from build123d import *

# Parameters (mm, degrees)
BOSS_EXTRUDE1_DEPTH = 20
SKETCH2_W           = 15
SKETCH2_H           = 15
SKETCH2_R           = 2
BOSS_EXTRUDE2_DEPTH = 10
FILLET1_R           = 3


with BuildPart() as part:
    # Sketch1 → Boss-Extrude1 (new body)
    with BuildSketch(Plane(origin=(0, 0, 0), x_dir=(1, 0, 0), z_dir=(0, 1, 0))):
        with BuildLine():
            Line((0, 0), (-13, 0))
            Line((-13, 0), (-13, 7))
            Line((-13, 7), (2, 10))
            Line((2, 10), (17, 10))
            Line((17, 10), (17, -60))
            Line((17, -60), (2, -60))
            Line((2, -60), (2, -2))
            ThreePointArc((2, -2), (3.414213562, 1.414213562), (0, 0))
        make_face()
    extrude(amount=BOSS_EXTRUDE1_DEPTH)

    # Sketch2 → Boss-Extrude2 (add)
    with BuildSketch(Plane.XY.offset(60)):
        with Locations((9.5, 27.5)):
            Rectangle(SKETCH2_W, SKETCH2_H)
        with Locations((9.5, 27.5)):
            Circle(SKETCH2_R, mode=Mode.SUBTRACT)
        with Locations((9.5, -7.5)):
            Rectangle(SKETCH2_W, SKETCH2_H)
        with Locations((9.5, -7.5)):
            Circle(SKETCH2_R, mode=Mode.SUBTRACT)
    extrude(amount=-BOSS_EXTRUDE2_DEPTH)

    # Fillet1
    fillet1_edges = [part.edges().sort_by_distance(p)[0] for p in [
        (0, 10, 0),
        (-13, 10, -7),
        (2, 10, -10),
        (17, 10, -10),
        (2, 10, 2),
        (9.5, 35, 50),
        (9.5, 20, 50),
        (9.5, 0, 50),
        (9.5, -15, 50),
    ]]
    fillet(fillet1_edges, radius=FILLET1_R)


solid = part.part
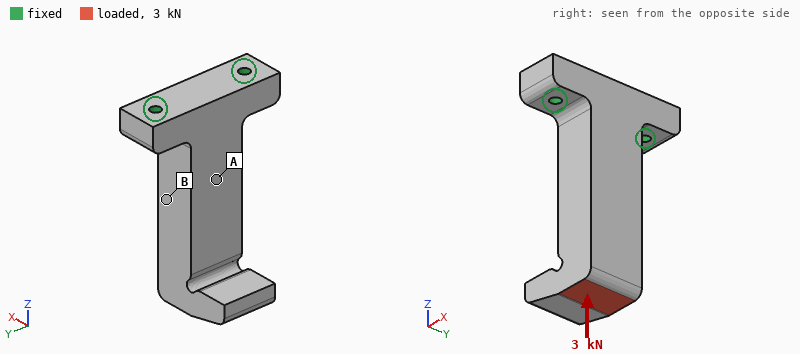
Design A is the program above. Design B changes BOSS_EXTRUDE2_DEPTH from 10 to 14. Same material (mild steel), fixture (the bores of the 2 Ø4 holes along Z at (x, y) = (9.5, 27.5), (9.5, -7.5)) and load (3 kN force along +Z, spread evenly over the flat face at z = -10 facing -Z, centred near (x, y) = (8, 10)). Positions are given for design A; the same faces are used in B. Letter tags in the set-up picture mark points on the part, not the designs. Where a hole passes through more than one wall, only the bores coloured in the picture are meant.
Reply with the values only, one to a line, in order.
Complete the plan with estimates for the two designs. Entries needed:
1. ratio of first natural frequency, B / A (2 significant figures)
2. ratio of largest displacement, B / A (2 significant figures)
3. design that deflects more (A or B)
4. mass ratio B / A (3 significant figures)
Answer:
1.3
0.80
A
1.06
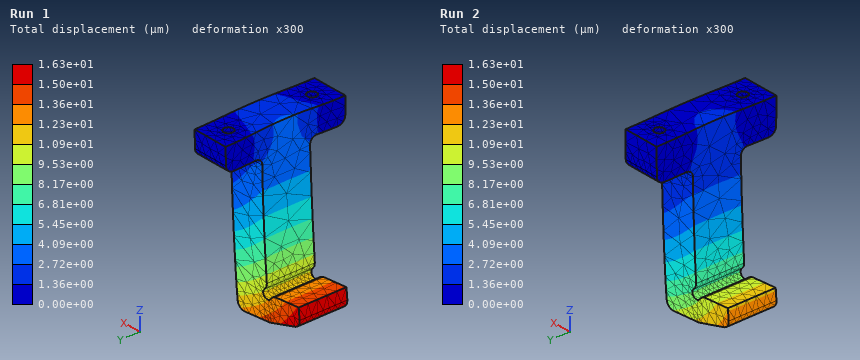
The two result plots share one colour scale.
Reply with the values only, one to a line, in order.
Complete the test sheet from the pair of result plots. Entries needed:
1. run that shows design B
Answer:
Run 2
